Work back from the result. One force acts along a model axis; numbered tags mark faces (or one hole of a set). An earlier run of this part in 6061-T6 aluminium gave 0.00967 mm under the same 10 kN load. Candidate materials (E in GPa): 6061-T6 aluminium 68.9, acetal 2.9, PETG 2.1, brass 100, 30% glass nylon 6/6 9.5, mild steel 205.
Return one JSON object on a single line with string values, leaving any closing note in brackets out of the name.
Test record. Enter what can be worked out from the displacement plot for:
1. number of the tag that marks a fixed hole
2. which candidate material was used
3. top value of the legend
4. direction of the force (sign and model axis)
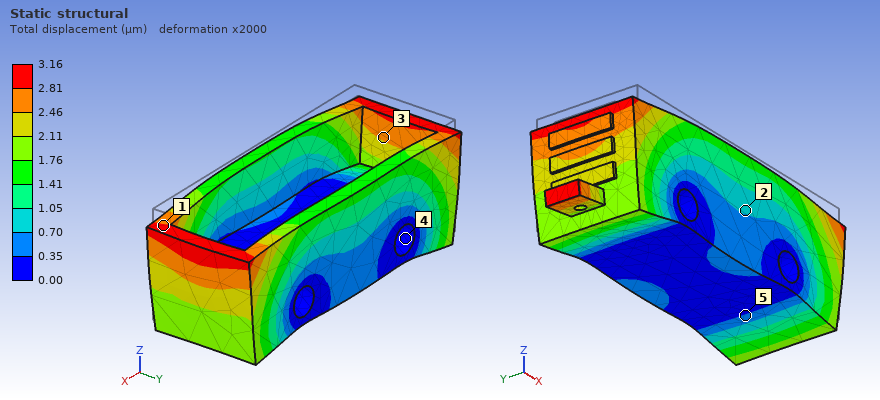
{"number of the tag that marks a fixed hole": "4", "which candidate material was used": "mild steel", "top value of the legend": "3.16 µm", "direction of the force": "-Z"}
